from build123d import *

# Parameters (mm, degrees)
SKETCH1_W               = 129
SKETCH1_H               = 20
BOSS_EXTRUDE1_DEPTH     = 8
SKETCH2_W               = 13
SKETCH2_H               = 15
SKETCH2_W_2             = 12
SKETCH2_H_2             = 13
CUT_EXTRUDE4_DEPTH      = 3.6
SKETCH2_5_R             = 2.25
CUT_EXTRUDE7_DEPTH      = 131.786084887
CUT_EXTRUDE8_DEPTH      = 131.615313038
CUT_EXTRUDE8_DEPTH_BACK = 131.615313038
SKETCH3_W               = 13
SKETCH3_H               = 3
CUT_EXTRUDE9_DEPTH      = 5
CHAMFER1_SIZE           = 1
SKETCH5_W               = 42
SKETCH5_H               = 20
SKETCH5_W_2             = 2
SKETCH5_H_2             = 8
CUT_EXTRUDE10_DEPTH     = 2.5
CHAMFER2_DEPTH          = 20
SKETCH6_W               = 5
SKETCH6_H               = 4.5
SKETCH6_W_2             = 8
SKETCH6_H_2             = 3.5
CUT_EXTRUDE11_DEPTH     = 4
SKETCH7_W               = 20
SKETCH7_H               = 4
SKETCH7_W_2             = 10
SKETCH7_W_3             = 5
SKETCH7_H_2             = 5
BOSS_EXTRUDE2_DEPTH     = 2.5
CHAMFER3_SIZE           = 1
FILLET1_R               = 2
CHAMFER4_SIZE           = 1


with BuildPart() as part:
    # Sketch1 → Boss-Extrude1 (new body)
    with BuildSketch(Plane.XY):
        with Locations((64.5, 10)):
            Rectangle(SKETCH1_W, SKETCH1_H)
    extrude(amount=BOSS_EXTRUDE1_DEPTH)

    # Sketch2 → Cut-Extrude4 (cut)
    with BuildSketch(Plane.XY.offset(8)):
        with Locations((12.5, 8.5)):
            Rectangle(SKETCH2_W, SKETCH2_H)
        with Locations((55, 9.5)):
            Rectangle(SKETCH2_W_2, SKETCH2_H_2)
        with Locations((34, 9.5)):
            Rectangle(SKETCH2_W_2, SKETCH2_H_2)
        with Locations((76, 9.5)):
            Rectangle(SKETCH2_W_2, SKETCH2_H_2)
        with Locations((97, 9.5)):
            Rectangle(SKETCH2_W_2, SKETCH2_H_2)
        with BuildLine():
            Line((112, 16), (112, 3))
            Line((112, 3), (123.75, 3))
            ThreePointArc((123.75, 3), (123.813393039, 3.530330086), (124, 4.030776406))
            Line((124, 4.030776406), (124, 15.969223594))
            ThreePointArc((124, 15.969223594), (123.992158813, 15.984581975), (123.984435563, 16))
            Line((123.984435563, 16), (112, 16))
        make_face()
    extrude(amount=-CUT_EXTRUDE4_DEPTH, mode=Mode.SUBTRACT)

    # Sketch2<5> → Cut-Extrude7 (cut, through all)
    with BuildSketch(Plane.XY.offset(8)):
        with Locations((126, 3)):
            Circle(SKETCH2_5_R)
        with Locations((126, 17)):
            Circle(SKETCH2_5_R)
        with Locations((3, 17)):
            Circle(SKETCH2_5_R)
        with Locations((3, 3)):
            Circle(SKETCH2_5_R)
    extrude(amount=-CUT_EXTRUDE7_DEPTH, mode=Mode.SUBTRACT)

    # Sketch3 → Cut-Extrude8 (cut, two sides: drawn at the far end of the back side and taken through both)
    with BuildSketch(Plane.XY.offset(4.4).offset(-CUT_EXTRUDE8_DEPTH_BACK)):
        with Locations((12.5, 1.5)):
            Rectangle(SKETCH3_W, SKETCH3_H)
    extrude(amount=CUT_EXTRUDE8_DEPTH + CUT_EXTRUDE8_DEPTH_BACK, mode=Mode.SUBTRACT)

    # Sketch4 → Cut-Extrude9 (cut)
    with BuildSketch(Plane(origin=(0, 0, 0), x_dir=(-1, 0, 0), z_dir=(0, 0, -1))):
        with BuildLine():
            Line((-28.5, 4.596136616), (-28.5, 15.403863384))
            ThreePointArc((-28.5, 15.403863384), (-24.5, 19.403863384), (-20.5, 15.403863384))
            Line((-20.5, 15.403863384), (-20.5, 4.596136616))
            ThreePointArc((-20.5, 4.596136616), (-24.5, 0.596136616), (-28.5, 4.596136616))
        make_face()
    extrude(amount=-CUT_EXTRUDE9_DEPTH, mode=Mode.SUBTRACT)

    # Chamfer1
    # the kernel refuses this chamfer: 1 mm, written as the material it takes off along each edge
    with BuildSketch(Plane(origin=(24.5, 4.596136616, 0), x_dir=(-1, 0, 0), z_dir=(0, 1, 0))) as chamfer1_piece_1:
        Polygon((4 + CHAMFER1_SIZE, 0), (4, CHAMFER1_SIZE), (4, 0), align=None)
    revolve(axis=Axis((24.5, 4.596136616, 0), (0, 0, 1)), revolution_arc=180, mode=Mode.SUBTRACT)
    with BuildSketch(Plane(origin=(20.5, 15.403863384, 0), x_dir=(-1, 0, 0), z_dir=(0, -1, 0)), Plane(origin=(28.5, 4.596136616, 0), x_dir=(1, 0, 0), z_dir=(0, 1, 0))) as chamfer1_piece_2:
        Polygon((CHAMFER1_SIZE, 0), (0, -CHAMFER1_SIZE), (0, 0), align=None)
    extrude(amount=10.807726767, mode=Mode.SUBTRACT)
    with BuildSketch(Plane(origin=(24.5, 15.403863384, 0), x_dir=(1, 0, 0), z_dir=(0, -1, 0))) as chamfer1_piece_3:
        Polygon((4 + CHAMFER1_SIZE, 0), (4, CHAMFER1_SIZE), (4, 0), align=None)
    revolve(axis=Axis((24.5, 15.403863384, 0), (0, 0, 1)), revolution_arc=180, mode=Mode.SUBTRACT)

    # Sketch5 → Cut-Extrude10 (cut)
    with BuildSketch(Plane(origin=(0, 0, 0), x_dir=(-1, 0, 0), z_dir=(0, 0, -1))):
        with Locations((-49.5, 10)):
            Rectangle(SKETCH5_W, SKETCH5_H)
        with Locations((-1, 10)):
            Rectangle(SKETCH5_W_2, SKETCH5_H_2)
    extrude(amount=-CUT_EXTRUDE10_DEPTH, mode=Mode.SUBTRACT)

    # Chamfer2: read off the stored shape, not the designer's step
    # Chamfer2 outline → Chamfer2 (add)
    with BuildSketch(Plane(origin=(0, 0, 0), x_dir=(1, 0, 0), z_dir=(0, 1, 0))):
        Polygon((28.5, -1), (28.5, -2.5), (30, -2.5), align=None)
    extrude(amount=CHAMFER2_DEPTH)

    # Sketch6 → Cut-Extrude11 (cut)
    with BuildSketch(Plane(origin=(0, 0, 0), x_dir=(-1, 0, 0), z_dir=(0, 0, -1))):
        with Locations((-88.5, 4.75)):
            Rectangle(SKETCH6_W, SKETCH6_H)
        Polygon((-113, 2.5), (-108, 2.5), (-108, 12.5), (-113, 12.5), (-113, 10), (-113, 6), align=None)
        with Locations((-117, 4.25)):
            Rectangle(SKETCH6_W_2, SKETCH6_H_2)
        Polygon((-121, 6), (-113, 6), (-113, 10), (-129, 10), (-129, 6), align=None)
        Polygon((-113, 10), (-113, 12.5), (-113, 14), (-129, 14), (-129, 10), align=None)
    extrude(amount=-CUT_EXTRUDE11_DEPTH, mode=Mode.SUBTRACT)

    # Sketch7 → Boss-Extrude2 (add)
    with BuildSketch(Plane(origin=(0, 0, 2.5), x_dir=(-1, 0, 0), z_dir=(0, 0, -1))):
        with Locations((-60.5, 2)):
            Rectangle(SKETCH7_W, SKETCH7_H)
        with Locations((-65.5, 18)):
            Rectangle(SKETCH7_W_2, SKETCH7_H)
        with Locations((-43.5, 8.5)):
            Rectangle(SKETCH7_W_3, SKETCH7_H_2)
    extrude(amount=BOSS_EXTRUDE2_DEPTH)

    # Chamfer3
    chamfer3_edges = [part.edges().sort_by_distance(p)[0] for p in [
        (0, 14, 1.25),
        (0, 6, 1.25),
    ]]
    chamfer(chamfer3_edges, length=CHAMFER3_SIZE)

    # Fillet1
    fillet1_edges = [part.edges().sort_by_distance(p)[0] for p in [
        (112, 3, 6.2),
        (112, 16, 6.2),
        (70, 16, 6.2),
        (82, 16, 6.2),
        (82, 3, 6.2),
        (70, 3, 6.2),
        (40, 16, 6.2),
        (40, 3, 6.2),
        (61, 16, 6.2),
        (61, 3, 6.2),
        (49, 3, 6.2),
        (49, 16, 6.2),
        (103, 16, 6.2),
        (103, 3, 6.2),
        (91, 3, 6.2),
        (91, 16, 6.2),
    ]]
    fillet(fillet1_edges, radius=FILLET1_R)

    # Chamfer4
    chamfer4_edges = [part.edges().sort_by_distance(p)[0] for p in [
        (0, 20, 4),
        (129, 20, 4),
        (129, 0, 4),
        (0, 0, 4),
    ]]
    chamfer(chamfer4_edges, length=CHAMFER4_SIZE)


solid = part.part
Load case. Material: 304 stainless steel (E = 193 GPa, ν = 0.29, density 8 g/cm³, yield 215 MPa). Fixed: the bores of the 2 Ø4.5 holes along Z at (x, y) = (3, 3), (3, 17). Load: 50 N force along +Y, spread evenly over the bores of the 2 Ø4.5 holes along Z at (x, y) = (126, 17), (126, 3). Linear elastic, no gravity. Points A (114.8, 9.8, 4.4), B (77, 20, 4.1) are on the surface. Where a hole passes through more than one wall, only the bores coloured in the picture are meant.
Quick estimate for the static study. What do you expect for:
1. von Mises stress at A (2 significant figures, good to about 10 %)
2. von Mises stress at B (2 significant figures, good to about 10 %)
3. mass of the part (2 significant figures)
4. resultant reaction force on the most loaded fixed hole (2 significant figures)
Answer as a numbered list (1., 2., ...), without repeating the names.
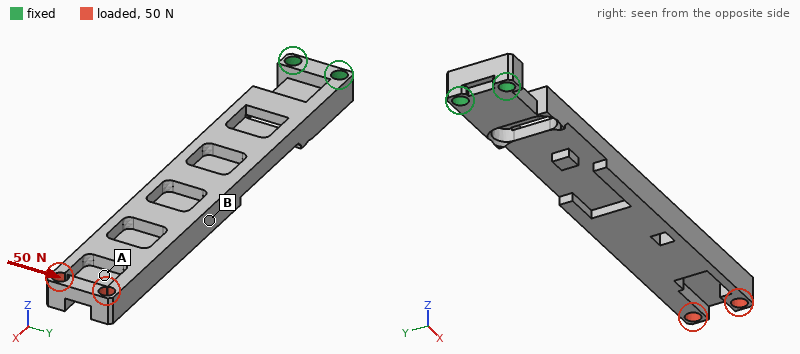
1. 8.9 MPa
2. 5.1 MPa
3. 100 g
4. 440 N
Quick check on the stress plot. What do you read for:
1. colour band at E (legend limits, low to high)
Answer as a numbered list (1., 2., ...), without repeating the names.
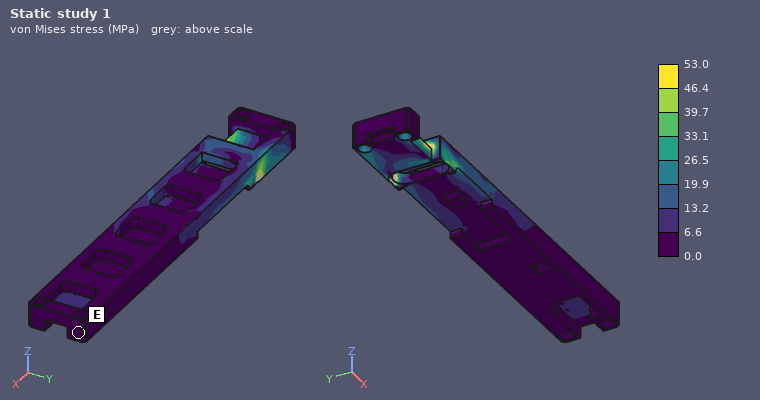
1. 0.0 to 6.6 MPa
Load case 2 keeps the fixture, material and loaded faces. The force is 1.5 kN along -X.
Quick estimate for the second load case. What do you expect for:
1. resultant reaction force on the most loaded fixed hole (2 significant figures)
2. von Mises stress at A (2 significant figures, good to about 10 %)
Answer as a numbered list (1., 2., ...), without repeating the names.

1. 800 N
2. 52 MPa
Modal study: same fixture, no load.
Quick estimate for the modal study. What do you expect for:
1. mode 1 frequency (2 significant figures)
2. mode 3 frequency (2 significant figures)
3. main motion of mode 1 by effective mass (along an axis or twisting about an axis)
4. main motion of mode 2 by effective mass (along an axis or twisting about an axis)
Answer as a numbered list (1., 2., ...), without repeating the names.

1. 210 Hz
2. 1800 Hz
3. along Z
4. along Y
